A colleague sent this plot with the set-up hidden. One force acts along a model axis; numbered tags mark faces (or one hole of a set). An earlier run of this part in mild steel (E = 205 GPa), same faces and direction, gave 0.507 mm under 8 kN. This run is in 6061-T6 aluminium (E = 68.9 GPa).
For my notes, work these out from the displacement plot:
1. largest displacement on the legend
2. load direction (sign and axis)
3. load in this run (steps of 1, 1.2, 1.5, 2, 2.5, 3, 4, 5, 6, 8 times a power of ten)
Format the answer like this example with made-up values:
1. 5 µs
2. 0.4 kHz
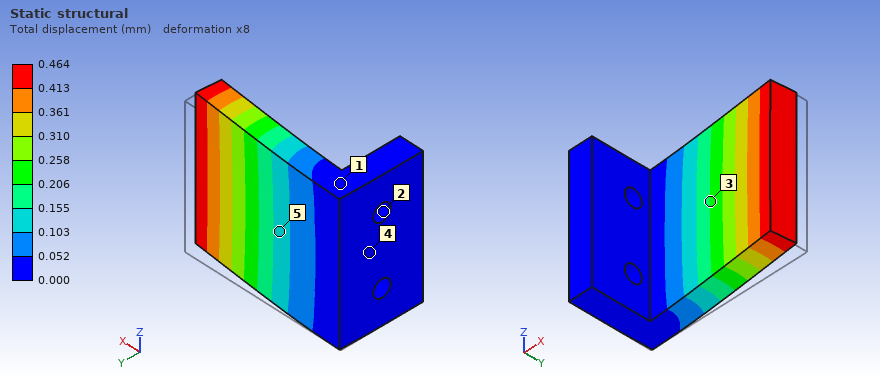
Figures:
1. 0.464 mm
2. -Y
3. 2.5 kN
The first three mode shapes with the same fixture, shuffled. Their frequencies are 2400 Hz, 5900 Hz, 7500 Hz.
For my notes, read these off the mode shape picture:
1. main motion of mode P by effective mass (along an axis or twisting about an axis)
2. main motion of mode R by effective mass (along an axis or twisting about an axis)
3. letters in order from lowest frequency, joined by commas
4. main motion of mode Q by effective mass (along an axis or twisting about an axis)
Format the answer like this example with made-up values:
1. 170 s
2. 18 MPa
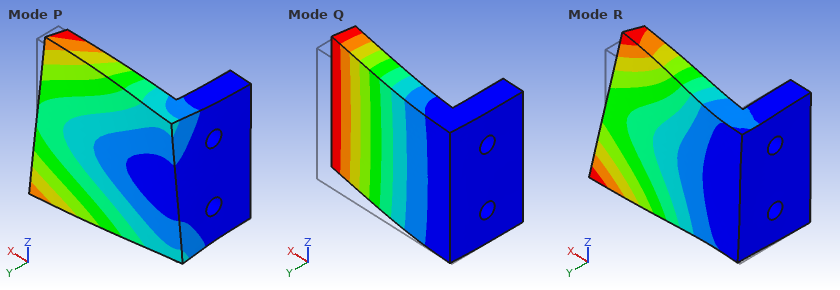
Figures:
1. along Z
2. along Z
3. Q, P, R
4. along Y
